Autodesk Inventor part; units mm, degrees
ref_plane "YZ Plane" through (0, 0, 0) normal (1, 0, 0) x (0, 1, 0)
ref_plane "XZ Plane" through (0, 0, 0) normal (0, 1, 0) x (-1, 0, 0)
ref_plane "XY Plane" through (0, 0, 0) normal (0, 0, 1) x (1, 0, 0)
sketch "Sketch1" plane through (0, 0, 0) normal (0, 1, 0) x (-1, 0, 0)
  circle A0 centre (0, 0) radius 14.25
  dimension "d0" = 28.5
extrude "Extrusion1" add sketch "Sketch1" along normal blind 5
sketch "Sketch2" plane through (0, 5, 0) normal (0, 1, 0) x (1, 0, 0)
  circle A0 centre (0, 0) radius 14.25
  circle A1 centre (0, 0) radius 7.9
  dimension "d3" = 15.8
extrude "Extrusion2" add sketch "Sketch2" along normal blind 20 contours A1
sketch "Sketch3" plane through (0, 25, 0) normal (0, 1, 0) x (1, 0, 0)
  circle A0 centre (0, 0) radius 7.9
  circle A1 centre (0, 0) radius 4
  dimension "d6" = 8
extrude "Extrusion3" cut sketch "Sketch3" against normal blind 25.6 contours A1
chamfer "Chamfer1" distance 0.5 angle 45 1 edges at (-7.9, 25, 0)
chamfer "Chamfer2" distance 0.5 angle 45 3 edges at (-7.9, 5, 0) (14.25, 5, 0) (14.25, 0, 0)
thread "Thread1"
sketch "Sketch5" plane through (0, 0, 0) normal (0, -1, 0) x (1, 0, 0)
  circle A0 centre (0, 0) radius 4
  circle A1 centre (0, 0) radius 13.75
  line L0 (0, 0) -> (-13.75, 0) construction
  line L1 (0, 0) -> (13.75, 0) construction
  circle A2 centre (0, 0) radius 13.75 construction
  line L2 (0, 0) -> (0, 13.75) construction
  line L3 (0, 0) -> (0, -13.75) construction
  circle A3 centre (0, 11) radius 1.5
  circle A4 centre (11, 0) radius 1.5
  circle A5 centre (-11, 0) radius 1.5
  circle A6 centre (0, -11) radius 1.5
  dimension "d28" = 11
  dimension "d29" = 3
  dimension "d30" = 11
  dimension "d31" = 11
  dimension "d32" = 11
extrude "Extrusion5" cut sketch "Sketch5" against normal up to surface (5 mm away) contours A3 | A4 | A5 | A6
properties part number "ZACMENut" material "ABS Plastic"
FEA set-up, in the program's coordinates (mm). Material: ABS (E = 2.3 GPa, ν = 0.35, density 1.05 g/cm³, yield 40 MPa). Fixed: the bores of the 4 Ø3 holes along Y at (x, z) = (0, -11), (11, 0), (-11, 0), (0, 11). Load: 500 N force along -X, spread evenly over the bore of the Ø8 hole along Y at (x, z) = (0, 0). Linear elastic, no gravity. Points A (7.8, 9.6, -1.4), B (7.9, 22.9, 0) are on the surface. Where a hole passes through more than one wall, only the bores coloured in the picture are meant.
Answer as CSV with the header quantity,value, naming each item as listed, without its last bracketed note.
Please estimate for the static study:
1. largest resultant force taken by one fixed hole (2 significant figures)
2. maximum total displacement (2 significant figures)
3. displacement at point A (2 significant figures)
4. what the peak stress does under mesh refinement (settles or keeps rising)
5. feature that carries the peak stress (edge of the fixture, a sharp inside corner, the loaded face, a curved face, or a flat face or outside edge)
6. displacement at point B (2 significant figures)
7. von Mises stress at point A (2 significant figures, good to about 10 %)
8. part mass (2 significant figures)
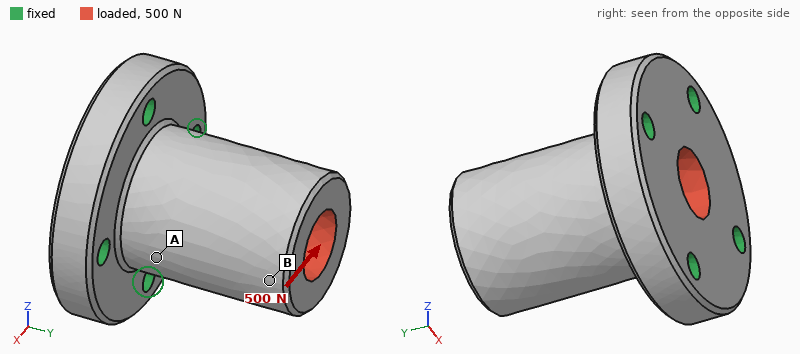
quantity,value
largest resultant force taken by one fixed hole,290 N
maximum total displacement,0.20 mm
displacement at point A,0.071 mm
what the peak stress does under mesh refinement,keeps rising
feature that carries the peak stress,a sharp inside corner
displacement at point B,0.18 mm
von Mises stress at point A,6.3 MPa
part mass,6.0 g
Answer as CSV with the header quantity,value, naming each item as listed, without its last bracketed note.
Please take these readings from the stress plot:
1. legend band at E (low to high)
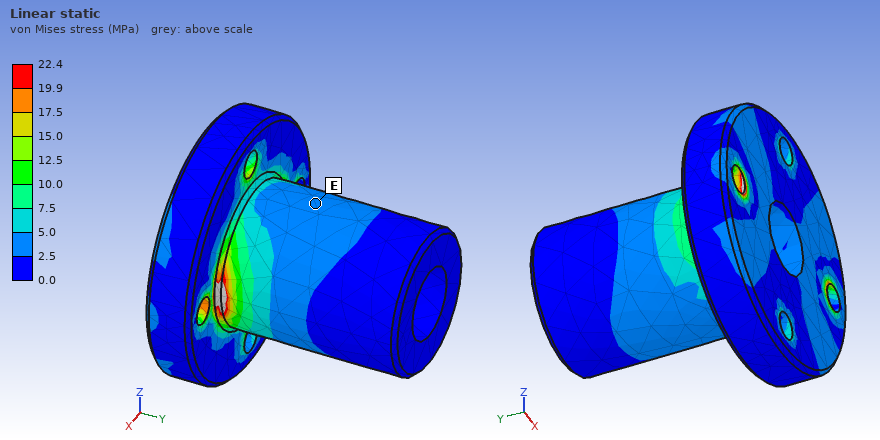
quantity,value
legend band at E,2.5 to 5.0 MPa
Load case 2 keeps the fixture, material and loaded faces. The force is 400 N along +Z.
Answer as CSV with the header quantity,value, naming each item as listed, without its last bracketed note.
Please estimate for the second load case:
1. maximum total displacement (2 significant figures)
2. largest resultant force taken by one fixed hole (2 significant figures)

quantity,value
maximum total displacement,0.16 mm
largest resultant force taken by one fixed hole,230 N
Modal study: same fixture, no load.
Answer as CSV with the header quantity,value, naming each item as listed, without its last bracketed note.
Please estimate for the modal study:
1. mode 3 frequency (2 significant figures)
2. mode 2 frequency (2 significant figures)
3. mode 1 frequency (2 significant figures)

quantity,value
mode 3 frequency,10 kHz
mode 2 frequency,4900 Hz
mode 1 frequency,4900 Hz
